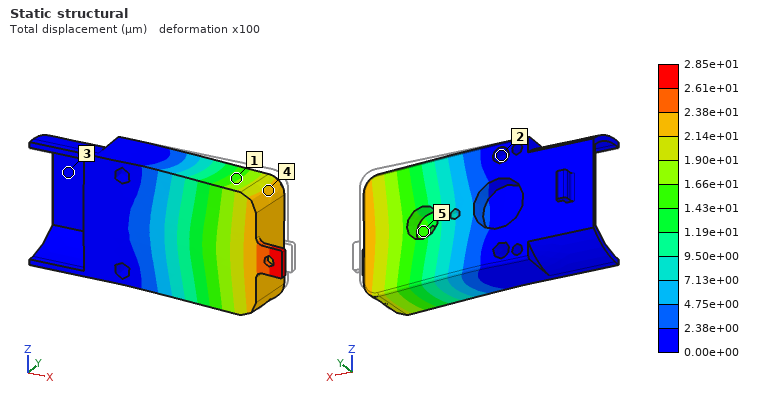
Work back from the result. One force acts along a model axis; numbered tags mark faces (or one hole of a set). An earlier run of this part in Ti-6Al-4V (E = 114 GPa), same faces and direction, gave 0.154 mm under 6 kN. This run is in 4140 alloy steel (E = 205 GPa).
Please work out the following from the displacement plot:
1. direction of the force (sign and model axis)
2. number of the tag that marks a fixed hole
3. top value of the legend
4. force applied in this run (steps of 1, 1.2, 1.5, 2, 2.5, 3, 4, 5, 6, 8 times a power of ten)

-Y
2
2.85e+01 µm
2 kN
